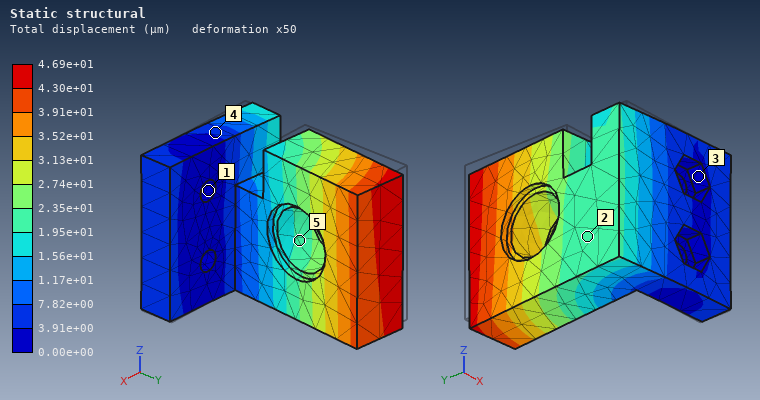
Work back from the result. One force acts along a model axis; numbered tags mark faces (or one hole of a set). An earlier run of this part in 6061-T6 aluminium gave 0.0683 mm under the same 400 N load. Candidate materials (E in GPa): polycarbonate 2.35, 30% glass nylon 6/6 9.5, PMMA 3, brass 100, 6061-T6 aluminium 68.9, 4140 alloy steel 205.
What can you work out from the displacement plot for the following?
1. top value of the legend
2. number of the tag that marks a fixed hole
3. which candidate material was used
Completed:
4.69e+01 µm
1
brass
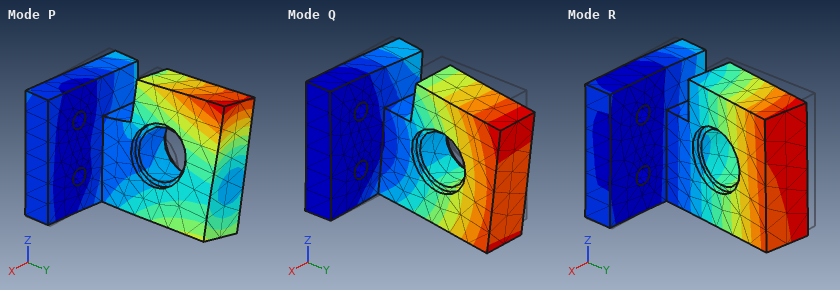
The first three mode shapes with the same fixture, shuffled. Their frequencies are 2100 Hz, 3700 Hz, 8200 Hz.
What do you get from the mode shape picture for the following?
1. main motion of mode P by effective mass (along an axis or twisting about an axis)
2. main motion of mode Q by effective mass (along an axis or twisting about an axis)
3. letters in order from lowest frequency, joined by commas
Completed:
along Y
along Z
R, Q, P
